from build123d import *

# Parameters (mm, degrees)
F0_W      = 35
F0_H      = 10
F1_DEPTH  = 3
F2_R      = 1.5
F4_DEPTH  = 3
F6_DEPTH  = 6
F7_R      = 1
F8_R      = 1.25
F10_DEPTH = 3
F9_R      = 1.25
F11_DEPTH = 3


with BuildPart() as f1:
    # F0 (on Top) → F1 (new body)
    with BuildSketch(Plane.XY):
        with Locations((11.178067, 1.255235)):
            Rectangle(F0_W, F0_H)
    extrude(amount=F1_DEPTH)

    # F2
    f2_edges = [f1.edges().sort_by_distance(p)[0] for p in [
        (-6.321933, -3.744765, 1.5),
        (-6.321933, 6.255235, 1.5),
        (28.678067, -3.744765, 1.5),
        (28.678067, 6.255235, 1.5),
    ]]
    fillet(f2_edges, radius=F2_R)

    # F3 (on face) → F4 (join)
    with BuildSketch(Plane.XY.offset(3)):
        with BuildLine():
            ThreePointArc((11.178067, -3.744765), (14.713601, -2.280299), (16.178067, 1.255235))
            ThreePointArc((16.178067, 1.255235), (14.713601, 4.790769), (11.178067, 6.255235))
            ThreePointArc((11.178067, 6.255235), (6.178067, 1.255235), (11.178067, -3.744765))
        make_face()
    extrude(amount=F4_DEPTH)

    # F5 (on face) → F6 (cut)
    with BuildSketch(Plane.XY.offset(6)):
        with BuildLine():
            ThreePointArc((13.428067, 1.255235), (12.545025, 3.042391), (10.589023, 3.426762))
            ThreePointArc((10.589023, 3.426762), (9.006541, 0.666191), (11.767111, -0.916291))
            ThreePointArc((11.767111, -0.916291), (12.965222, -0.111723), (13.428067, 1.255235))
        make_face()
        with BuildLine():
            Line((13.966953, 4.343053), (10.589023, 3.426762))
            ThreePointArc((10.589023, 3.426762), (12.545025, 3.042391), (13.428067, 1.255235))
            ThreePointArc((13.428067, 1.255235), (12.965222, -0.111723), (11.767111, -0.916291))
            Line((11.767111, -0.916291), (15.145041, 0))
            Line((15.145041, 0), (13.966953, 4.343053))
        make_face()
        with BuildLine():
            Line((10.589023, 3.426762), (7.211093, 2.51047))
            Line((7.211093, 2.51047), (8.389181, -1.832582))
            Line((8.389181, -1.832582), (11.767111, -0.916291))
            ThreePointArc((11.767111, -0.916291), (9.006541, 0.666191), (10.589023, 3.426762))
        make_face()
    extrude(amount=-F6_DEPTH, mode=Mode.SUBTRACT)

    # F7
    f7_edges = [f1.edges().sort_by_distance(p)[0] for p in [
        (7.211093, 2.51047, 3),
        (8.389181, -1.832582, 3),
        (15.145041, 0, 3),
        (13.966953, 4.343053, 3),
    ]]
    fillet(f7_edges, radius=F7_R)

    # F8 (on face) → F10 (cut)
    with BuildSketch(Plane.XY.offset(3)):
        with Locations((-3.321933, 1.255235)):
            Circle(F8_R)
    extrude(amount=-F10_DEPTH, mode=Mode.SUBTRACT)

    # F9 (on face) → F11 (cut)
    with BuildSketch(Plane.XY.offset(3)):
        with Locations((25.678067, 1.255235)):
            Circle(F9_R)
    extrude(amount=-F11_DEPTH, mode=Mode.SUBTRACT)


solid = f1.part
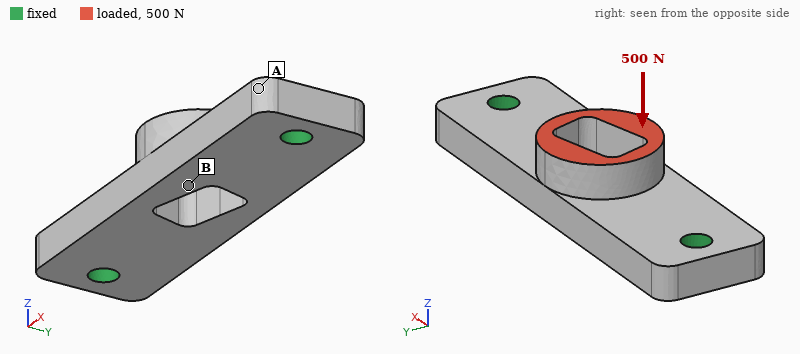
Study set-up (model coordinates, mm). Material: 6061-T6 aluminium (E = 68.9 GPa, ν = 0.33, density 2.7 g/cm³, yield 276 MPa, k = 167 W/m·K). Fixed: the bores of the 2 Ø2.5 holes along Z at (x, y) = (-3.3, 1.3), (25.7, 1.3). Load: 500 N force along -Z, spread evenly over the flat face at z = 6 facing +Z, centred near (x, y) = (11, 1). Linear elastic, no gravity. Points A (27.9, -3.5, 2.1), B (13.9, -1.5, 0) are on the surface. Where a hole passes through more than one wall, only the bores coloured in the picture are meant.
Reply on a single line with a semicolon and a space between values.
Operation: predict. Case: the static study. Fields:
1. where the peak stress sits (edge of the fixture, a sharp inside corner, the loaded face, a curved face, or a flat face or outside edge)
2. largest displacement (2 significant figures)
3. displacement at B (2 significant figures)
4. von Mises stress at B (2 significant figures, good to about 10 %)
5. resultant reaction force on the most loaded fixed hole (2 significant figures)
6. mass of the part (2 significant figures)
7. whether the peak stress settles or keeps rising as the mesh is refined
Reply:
edge of the fixture; 35 µm; 31 µm; 59 MPa; 270 N; 2.9 g; keeps rising
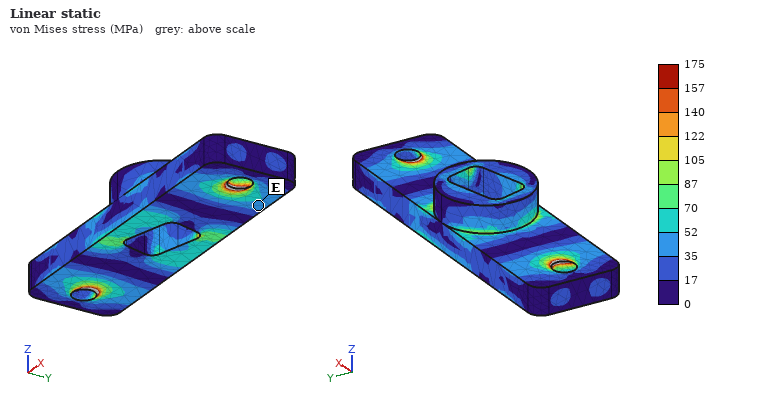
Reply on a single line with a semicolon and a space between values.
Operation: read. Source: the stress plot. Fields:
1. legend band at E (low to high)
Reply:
35 to 52 MPa
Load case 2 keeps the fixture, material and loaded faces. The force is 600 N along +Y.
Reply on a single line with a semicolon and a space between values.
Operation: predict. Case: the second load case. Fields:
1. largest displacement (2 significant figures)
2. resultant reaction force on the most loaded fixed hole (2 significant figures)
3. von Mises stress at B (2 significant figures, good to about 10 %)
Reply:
65 µm; 300 N; 51 MPa
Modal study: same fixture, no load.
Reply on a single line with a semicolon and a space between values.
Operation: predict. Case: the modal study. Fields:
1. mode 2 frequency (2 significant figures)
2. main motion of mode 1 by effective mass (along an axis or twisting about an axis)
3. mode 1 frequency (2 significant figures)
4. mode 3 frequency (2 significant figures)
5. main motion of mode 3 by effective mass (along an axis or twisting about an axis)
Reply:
22 kHz; along Z; 18 kHz; 31 kHz; along Y
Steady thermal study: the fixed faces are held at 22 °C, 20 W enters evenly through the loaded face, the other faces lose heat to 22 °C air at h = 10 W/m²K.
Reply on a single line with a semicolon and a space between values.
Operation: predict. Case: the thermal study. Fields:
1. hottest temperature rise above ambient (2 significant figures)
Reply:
33 K
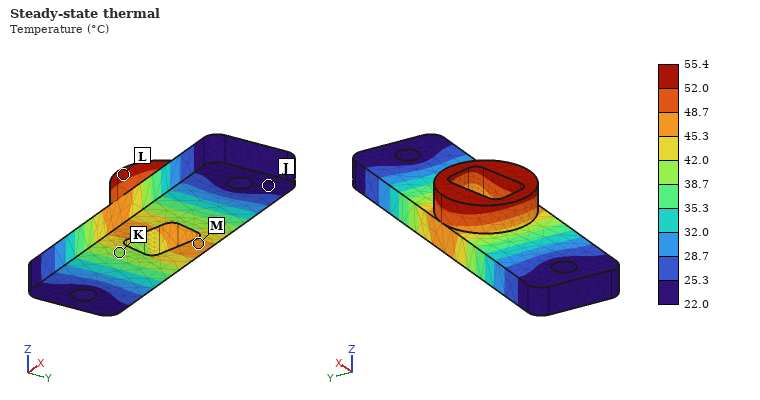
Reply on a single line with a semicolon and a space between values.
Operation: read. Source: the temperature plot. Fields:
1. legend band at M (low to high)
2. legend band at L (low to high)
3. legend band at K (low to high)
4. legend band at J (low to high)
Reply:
45.3 to 48.7 °C; 52.0 to 55.4 °C; 38.7 to 42.0 °C; 22.0 to 25.3 °C
